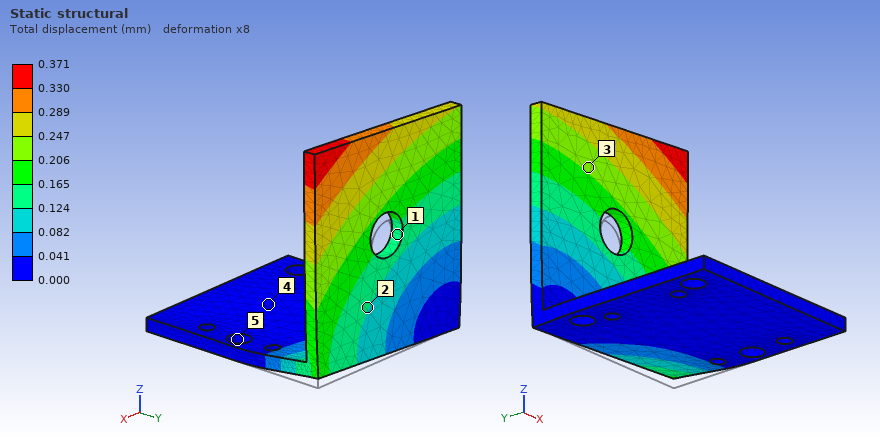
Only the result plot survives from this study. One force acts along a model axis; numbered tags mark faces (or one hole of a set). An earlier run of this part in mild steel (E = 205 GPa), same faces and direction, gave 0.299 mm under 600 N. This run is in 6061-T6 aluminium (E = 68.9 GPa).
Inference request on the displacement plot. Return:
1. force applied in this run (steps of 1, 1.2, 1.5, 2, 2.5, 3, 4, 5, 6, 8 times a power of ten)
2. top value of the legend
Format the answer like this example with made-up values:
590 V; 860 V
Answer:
250 N; 0.371 mm
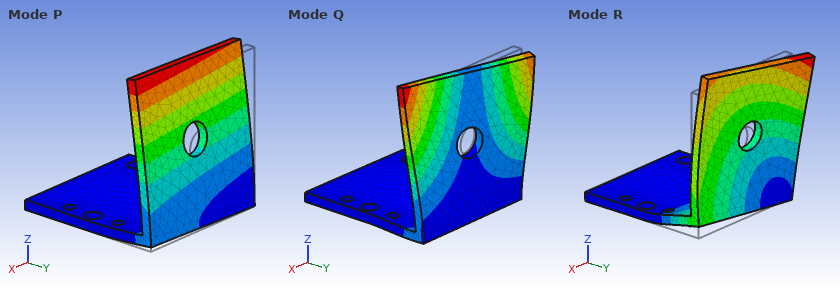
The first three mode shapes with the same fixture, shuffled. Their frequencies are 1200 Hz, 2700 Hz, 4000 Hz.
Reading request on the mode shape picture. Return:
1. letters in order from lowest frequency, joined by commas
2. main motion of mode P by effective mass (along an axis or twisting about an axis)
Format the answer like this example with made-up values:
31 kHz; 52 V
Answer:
P, R, Q; along Y
